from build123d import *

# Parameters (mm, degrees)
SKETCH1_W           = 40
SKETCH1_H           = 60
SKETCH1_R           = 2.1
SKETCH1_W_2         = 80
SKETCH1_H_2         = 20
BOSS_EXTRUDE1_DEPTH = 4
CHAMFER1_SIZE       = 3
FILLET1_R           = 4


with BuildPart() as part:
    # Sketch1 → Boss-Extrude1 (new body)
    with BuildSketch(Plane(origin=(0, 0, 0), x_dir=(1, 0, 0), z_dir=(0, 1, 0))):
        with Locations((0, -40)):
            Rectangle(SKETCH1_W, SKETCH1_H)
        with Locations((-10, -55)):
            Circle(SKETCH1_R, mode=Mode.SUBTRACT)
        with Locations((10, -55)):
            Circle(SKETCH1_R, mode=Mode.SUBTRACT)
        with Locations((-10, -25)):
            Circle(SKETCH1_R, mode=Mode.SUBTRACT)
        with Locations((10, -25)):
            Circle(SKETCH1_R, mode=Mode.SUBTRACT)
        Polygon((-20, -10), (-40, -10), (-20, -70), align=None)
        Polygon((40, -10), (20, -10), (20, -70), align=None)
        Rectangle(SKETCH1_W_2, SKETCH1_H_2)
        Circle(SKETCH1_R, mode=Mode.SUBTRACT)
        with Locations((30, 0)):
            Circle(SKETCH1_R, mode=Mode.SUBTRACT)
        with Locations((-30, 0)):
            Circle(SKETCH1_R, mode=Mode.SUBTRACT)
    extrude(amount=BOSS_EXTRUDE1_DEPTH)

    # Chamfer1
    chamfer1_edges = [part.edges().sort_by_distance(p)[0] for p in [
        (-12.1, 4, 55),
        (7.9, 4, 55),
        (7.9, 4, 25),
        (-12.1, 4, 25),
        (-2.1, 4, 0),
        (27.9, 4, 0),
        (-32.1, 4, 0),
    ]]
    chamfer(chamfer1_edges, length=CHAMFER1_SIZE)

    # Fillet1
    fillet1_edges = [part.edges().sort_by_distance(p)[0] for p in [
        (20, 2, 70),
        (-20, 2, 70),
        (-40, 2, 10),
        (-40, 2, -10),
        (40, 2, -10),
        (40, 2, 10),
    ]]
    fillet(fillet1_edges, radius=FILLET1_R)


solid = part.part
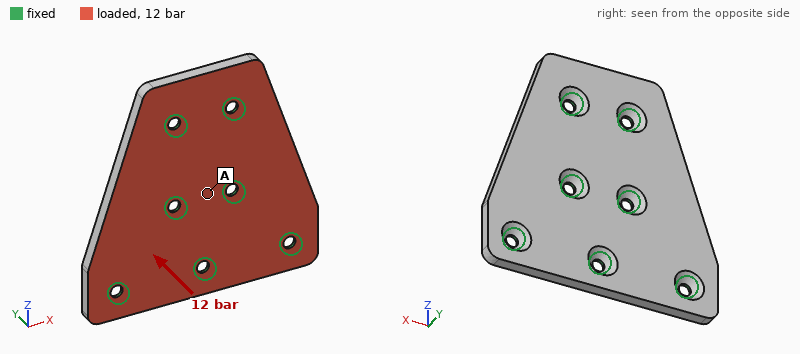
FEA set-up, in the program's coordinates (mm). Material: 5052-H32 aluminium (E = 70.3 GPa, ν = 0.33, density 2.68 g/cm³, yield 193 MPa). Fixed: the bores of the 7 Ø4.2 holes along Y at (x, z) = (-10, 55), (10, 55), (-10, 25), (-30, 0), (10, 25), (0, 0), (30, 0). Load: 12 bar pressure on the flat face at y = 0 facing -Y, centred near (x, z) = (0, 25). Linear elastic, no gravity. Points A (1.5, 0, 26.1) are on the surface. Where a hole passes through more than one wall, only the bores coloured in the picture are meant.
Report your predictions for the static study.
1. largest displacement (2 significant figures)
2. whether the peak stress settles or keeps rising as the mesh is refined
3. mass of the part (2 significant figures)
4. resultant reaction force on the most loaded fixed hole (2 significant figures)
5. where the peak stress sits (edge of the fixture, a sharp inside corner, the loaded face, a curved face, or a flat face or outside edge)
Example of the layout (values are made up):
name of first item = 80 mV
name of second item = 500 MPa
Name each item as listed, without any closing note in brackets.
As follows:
largest displacement = 0.11 mm
whether the peak stress settles or keeps rising as the mesh is refined = keeps rising
mass of the part = 53 g
resultant reaction force on the most loaded fixed hole = 1.2 kN
where the peak stress sits = edge of the fixture
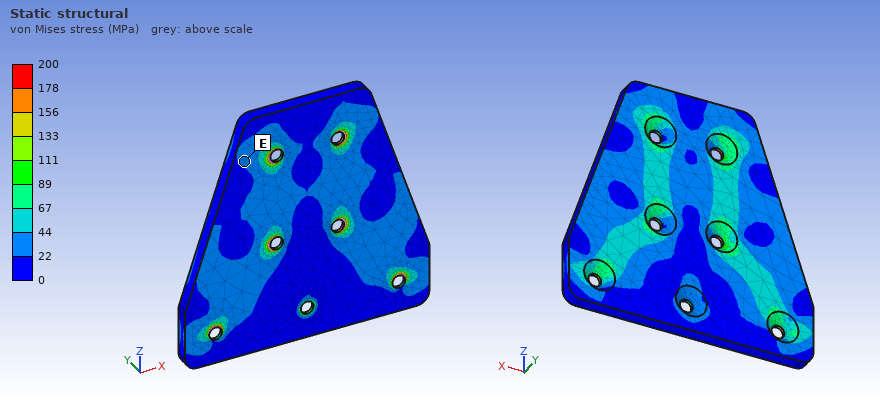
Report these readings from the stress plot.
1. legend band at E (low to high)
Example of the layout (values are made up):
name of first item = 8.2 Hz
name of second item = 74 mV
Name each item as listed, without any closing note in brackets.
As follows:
legend band at E = 22 to 44 MPa
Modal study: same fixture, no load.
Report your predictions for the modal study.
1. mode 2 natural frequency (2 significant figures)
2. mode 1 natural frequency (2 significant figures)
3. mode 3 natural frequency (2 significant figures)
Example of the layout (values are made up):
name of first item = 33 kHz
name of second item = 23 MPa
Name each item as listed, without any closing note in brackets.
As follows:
mode 2 natural frequency = 6500 Hz
mode 1 natural frequency = 6500 Hz
mode 3 natural frequency = 9600 Hz
